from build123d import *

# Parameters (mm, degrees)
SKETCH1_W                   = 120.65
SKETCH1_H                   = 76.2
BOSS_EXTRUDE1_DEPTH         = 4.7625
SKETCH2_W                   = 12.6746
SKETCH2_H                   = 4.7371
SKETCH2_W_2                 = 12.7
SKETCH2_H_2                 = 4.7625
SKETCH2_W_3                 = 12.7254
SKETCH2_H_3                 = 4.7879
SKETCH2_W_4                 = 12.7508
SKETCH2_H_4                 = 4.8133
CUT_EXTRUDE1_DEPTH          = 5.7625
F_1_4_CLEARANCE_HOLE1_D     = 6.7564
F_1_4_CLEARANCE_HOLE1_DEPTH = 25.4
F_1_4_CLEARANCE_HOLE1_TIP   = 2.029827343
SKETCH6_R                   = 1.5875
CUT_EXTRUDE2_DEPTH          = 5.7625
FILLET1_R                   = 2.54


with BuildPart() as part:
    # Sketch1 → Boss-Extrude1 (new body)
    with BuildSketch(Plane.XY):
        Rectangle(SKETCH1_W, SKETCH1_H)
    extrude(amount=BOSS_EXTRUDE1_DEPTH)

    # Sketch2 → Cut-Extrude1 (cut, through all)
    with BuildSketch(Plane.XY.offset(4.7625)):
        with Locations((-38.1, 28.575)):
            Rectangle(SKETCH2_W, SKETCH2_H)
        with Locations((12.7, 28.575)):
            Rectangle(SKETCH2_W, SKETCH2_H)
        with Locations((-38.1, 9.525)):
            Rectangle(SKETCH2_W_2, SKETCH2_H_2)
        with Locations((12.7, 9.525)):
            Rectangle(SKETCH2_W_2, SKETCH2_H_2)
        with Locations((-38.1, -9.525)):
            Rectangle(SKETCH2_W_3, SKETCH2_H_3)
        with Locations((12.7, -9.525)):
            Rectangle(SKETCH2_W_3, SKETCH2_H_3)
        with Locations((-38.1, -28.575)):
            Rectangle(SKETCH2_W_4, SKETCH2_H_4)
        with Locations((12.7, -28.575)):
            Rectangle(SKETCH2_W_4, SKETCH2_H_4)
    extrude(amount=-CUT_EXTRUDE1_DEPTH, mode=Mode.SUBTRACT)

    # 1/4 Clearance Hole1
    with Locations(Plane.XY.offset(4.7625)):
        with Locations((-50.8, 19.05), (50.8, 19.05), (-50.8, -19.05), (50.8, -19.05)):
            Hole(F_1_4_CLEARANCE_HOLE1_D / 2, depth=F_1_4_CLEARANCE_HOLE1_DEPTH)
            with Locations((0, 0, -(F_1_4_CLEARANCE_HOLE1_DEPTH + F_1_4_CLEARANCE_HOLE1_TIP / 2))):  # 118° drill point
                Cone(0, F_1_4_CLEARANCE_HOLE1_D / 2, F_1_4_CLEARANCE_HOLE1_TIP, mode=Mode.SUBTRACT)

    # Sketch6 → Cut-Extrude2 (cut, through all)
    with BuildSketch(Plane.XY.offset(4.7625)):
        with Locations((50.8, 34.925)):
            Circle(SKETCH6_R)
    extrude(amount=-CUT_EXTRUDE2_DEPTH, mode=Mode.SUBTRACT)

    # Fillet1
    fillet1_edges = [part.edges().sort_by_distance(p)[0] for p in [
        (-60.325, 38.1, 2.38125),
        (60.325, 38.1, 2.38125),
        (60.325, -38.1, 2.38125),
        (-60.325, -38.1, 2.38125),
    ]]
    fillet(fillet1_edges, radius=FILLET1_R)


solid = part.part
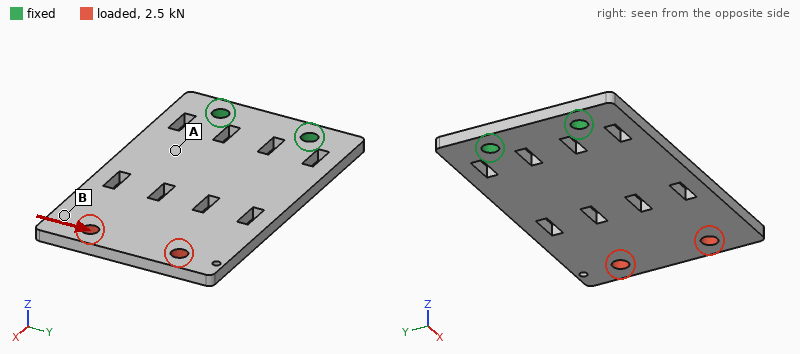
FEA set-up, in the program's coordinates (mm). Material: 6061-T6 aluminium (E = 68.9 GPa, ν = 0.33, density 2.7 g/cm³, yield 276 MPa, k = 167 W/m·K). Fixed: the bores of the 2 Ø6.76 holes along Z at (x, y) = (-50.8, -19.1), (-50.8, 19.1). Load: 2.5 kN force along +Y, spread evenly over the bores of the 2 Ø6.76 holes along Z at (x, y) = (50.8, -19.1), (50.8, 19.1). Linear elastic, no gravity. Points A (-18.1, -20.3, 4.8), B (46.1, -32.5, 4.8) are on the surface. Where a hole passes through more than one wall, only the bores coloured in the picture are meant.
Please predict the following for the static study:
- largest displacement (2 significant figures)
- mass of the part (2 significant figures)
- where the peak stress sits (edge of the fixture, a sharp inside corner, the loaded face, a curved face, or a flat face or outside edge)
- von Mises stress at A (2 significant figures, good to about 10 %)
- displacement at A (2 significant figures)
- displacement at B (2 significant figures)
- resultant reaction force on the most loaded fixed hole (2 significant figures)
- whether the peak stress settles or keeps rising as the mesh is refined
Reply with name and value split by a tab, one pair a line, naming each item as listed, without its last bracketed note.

largest displacement	0.22 mm
mass of the part	110 g
where the peak stress sits	edge of the fixture
von Mises stress at A	29 MPa
displacement at A	0.056 mm
displacement at B	0.19 mm
resultant reaction force on the most loaded fixed hole	5.9 kN
whether the peak stress settles or keeps rising as the mesh is refined	keeps rising
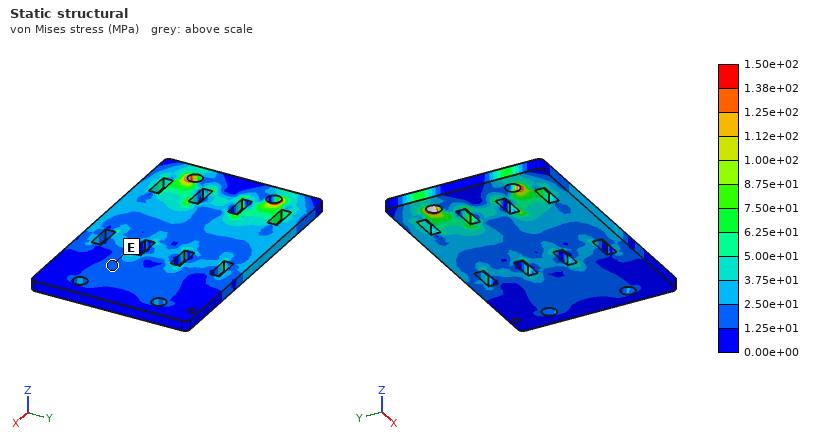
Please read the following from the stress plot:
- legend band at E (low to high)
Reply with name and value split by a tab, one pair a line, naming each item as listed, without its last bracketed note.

legend band at E	1.25e+01 to 2.50e+01 MPa
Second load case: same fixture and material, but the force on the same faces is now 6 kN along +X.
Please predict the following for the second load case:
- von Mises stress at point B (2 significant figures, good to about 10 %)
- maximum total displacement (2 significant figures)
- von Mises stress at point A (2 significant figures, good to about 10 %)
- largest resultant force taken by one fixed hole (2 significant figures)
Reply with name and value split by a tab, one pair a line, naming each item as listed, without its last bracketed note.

von Mises stress at point B	9.8 MPa
maximum total displacement	38 µm
von Mises stress at point A	20 MPa
largest resultant force taken by one fixed hole	3.0 kN
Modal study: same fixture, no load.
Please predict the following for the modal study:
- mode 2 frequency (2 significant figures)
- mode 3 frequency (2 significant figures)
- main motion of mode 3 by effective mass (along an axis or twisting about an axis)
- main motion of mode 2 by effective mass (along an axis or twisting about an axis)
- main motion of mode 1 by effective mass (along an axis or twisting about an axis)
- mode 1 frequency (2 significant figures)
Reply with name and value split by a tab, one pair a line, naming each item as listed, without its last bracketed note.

mode 2 frequency	970 Hz
mode 3 frequency	1900 Hz
main motion of mode 3 by effective mass	along Z
main motion of mode 2 by effective mass	twisting about X
main motion of mode 1 by effective mass	along Z
mode 1 frequency	300 Hz
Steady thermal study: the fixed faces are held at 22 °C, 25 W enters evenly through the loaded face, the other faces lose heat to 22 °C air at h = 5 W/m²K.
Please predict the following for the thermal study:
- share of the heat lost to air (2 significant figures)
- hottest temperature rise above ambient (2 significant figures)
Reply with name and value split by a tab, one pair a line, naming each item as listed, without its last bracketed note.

share of the heat lost to air	9.4 %
hottest temperature rise above ambient	48 K
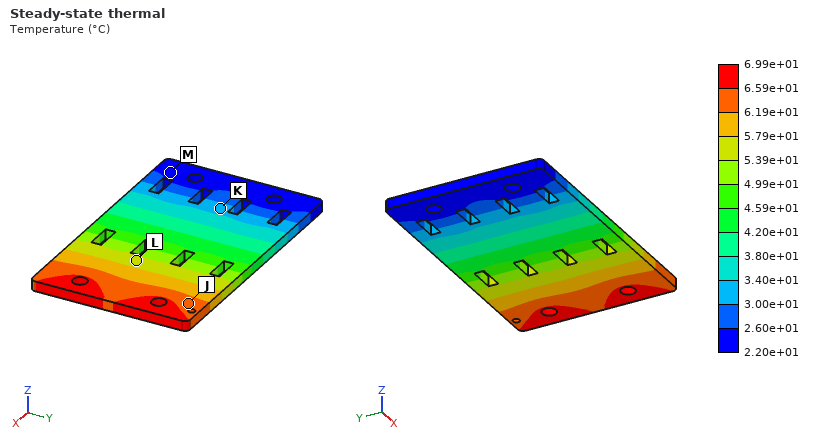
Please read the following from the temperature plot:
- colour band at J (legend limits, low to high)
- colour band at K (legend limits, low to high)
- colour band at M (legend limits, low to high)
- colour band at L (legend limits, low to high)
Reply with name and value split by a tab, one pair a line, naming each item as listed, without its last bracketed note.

colour band at J	6.19e+01 to 6.59e+01 °C
colour band at K	3.00e+01 to 3.40e+01 °C
colour band at M	2.20e+01 to 2.60e+01 °C
colour band at L	5.39e+01 to 5.79e+01 °C
